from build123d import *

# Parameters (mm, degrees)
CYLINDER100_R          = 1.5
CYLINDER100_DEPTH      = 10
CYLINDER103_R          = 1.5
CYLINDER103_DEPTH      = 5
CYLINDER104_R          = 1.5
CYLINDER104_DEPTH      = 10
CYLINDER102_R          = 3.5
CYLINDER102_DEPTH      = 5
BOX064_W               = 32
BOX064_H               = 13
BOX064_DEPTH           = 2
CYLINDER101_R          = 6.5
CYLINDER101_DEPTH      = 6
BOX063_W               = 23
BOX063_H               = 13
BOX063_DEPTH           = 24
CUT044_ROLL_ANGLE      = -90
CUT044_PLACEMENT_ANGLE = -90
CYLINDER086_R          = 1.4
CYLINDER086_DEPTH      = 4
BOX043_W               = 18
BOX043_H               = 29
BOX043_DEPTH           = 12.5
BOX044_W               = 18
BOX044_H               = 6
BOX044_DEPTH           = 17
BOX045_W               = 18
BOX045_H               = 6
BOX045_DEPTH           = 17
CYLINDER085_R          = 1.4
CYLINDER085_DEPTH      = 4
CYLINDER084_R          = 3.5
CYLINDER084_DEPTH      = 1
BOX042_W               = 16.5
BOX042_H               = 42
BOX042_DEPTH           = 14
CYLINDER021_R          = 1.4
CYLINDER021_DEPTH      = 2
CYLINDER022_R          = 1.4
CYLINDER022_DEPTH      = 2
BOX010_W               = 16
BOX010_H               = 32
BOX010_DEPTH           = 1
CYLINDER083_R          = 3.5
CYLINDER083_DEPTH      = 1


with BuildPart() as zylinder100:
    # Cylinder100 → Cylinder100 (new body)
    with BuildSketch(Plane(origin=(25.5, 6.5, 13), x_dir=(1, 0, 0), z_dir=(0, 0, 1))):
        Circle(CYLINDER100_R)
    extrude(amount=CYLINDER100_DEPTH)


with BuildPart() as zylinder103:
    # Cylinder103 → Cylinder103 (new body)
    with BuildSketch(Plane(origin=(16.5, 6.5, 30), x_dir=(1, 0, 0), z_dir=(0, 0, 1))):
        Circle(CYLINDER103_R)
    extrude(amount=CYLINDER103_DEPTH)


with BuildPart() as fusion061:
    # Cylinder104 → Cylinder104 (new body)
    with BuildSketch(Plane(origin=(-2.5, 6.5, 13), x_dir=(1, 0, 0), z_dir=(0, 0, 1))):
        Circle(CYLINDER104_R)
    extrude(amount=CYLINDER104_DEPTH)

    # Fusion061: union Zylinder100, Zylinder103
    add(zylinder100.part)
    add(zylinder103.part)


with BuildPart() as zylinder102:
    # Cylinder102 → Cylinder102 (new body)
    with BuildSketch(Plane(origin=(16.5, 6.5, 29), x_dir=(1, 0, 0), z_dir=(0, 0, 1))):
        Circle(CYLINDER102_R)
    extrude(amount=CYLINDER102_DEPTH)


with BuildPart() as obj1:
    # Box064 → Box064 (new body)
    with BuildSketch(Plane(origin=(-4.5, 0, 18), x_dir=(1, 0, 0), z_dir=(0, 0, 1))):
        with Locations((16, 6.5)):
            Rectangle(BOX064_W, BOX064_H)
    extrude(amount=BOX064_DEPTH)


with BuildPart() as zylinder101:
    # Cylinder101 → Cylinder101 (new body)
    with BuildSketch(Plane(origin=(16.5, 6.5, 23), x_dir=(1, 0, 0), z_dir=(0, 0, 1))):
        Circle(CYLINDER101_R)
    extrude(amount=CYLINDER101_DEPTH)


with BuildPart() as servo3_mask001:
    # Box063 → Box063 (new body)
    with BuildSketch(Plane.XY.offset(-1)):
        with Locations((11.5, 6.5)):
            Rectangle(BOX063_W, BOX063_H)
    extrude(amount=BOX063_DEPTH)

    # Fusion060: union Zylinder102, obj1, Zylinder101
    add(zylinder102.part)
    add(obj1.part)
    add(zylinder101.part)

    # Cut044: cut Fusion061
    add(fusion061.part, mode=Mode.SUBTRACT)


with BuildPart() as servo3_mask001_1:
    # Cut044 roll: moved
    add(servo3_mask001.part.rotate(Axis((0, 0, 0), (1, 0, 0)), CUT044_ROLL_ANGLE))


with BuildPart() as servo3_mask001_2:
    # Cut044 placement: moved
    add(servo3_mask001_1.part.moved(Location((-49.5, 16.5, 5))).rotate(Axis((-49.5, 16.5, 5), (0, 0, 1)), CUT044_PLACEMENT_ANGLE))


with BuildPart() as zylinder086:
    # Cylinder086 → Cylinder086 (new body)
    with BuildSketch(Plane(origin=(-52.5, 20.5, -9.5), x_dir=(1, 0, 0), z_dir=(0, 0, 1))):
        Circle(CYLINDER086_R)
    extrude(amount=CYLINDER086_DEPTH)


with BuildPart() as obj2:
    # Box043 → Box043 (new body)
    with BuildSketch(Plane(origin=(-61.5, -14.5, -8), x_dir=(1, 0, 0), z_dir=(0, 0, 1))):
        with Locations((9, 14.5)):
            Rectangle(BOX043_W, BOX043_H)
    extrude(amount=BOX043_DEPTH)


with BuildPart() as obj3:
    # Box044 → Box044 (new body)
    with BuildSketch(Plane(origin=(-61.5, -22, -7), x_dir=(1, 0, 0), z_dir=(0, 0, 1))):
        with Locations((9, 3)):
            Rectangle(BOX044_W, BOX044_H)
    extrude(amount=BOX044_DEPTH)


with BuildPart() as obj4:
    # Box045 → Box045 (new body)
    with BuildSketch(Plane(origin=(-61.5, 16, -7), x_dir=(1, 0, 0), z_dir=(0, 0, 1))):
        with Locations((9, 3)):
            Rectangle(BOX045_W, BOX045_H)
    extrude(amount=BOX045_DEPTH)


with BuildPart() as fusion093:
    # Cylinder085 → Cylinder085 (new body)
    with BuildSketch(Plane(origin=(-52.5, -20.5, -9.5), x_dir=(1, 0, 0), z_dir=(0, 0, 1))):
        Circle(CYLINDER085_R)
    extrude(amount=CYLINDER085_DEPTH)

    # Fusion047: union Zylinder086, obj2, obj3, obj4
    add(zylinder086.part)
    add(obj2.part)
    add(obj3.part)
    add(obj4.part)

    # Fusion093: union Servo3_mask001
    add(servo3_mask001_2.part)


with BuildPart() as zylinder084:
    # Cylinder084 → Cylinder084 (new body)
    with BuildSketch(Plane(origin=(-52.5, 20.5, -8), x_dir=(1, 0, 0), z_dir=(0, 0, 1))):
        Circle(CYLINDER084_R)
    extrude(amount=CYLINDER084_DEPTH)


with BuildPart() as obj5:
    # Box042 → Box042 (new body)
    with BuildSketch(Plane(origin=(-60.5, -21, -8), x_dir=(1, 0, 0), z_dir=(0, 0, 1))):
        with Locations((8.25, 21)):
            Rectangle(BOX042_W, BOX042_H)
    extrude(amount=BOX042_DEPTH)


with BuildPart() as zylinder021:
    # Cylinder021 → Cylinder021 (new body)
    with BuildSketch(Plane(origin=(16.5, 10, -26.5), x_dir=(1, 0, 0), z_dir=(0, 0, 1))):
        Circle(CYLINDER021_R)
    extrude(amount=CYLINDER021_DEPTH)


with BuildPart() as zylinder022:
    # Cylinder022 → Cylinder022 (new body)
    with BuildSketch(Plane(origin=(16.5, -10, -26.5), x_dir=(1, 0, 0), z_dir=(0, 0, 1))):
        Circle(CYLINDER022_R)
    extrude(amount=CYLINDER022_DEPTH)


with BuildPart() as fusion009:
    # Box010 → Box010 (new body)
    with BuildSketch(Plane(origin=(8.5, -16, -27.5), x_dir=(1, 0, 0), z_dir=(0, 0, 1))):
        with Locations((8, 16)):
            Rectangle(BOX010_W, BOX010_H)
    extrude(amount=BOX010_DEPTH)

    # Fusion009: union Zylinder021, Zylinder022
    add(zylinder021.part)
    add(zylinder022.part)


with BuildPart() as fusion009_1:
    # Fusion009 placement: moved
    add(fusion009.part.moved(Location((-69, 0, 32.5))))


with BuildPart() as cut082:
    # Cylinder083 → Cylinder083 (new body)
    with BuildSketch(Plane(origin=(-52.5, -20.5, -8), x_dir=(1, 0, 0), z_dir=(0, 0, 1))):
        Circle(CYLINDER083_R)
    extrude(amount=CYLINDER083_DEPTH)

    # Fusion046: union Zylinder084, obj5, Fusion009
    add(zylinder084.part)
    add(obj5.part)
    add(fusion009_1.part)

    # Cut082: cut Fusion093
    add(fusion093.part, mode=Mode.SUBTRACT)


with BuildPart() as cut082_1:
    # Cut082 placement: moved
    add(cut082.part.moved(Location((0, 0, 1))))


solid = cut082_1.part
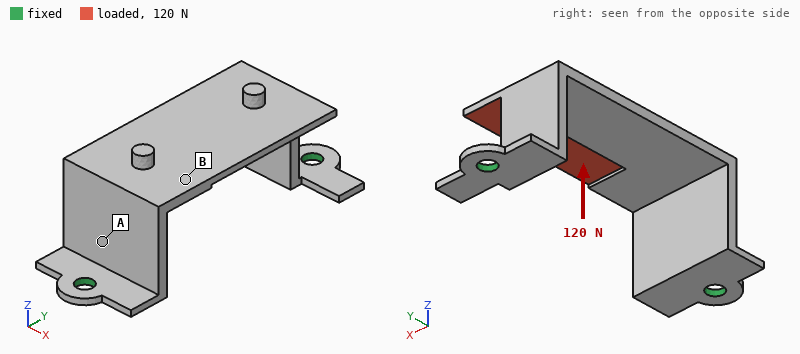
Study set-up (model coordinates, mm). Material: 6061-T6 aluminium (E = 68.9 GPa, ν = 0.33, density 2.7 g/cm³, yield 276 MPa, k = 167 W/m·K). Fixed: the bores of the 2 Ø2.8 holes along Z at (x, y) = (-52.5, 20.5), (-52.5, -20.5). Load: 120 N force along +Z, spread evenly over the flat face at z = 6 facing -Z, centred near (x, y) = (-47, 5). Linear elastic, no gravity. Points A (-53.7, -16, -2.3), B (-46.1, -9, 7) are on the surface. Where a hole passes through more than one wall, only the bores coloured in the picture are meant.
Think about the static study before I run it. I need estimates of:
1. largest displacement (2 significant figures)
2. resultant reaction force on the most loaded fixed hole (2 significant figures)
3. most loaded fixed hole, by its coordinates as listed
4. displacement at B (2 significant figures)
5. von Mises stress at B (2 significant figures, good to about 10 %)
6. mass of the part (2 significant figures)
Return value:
0.30 mm
85 N
(-52.5, 20.5)
0.17 mm
44 MPa
3.8 g
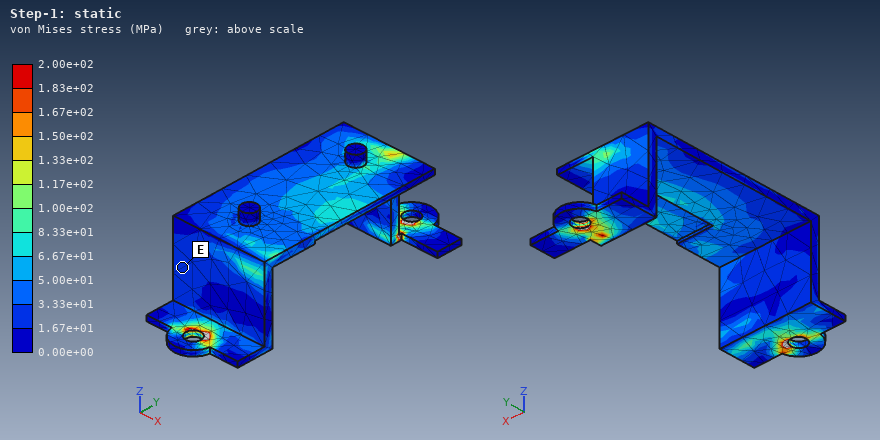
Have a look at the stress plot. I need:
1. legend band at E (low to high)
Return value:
1.67e+01 to 3.33e+01 MPa
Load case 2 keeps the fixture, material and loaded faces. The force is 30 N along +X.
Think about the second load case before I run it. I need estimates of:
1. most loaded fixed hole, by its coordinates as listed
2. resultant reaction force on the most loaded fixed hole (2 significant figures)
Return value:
(-52.5, 20.5)
17 N
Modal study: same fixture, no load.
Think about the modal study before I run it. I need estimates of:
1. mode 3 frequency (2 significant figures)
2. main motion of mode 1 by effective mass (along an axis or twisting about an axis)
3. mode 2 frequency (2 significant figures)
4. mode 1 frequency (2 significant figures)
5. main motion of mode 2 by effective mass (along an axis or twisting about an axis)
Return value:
3900 Hz
along X
2800 Hz
1900 Hz
along Y
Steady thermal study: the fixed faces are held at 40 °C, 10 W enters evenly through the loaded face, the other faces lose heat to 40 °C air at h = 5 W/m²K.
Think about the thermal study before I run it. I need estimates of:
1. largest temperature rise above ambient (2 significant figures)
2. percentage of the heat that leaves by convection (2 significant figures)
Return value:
55 K
3.1 %
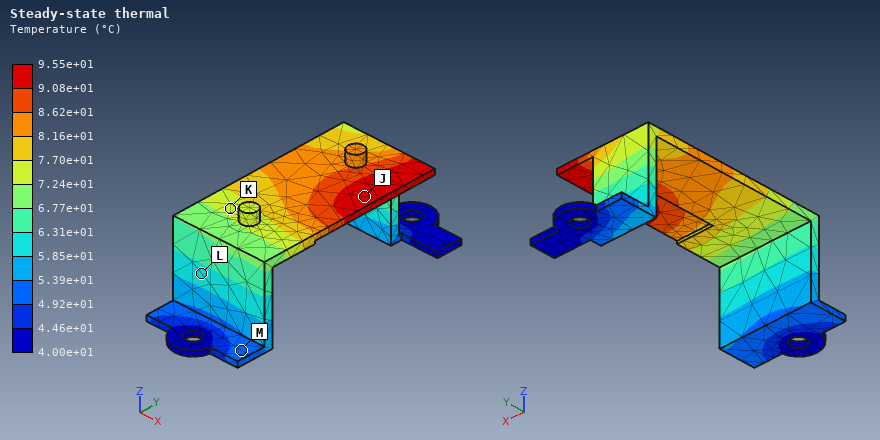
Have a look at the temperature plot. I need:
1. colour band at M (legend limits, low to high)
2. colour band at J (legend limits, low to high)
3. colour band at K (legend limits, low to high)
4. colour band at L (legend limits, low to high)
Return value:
4.92e+01 to 5.39e+01 °C
9.08e+01 to 9.55e+01 °C
7.24e+01 to 7.70e+01 °C
5.85e+01 to 6.31e+01 °C
